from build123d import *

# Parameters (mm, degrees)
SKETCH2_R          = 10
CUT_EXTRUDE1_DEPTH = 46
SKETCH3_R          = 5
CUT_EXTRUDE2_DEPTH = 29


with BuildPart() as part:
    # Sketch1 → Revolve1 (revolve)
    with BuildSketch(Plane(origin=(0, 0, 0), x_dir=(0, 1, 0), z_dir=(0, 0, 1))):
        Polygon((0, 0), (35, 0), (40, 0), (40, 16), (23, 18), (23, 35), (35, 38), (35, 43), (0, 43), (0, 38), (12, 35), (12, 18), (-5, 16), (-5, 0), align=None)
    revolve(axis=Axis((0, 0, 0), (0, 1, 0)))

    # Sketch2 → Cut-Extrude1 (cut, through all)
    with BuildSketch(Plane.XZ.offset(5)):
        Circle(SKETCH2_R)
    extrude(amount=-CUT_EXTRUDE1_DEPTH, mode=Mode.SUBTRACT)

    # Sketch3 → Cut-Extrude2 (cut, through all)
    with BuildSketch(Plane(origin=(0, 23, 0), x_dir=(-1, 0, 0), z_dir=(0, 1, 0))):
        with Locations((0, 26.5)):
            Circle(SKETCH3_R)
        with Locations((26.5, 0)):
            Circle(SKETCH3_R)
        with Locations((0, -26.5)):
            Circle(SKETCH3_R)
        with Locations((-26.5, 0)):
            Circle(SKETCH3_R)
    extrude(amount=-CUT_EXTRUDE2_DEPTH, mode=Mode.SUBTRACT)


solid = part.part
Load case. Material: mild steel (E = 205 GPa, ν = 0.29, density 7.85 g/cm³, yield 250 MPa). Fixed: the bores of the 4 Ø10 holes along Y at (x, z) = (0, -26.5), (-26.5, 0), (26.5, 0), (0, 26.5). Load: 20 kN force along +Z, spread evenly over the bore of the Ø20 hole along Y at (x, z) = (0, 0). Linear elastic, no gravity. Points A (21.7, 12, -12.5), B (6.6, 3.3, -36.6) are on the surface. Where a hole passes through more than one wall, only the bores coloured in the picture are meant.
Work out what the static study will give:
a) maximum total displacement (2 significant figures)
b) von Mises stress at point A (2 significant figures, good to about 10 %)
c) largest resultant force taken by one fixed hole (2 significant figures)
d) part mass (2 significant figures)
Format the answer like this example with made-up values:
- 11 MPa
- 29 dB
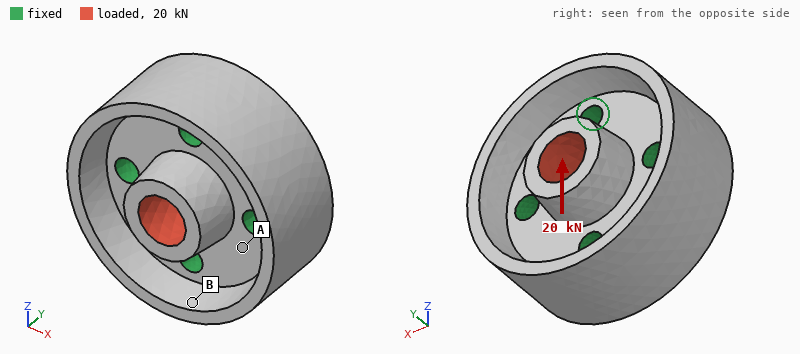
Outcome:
- 5.0 µm
- 8.1 MPa
- 6.2 kN
- 910 g
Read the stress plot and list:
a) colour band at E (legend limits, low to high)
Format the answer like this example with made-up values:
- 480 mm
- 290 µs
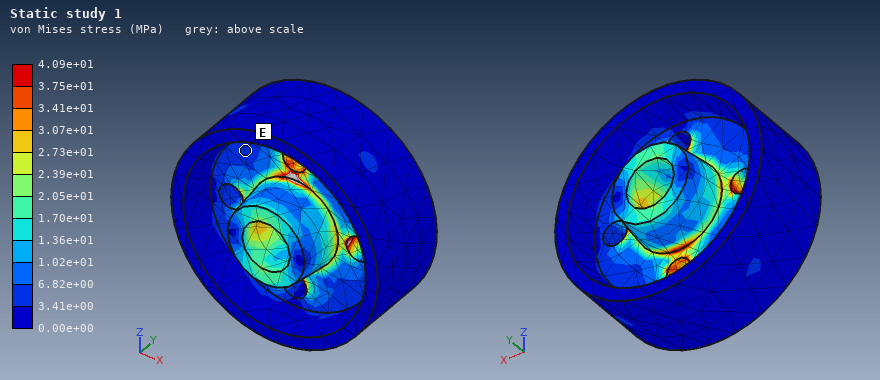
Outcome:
- 3.41e+00 to 6.82e+00 MPa
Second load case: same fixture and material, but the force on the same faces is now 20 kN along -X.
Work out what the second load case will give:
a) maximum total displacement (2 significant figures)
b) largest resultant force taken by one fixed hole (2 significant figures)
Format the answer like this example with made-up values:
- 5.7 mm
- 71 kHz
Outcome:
- 5.0 µm
- 6.2 kN
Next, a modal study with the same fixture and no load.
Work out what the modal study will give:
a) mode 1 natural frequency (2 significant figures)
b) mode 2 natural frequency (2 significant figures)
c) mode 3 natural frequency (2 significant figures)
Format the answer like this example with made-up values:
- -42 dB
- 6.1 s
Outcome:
- 10 kHz
- 13 kHz
- 13 kHz
